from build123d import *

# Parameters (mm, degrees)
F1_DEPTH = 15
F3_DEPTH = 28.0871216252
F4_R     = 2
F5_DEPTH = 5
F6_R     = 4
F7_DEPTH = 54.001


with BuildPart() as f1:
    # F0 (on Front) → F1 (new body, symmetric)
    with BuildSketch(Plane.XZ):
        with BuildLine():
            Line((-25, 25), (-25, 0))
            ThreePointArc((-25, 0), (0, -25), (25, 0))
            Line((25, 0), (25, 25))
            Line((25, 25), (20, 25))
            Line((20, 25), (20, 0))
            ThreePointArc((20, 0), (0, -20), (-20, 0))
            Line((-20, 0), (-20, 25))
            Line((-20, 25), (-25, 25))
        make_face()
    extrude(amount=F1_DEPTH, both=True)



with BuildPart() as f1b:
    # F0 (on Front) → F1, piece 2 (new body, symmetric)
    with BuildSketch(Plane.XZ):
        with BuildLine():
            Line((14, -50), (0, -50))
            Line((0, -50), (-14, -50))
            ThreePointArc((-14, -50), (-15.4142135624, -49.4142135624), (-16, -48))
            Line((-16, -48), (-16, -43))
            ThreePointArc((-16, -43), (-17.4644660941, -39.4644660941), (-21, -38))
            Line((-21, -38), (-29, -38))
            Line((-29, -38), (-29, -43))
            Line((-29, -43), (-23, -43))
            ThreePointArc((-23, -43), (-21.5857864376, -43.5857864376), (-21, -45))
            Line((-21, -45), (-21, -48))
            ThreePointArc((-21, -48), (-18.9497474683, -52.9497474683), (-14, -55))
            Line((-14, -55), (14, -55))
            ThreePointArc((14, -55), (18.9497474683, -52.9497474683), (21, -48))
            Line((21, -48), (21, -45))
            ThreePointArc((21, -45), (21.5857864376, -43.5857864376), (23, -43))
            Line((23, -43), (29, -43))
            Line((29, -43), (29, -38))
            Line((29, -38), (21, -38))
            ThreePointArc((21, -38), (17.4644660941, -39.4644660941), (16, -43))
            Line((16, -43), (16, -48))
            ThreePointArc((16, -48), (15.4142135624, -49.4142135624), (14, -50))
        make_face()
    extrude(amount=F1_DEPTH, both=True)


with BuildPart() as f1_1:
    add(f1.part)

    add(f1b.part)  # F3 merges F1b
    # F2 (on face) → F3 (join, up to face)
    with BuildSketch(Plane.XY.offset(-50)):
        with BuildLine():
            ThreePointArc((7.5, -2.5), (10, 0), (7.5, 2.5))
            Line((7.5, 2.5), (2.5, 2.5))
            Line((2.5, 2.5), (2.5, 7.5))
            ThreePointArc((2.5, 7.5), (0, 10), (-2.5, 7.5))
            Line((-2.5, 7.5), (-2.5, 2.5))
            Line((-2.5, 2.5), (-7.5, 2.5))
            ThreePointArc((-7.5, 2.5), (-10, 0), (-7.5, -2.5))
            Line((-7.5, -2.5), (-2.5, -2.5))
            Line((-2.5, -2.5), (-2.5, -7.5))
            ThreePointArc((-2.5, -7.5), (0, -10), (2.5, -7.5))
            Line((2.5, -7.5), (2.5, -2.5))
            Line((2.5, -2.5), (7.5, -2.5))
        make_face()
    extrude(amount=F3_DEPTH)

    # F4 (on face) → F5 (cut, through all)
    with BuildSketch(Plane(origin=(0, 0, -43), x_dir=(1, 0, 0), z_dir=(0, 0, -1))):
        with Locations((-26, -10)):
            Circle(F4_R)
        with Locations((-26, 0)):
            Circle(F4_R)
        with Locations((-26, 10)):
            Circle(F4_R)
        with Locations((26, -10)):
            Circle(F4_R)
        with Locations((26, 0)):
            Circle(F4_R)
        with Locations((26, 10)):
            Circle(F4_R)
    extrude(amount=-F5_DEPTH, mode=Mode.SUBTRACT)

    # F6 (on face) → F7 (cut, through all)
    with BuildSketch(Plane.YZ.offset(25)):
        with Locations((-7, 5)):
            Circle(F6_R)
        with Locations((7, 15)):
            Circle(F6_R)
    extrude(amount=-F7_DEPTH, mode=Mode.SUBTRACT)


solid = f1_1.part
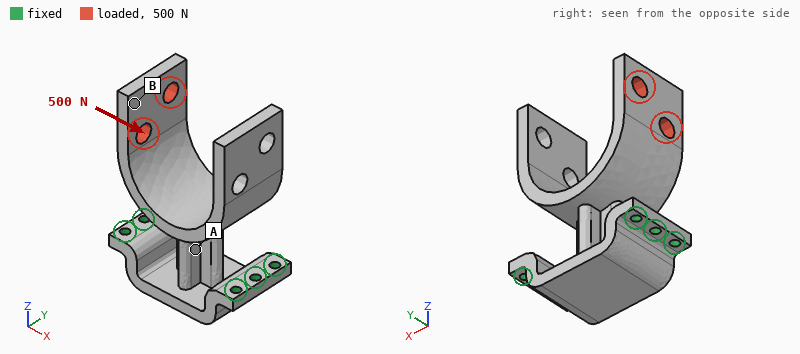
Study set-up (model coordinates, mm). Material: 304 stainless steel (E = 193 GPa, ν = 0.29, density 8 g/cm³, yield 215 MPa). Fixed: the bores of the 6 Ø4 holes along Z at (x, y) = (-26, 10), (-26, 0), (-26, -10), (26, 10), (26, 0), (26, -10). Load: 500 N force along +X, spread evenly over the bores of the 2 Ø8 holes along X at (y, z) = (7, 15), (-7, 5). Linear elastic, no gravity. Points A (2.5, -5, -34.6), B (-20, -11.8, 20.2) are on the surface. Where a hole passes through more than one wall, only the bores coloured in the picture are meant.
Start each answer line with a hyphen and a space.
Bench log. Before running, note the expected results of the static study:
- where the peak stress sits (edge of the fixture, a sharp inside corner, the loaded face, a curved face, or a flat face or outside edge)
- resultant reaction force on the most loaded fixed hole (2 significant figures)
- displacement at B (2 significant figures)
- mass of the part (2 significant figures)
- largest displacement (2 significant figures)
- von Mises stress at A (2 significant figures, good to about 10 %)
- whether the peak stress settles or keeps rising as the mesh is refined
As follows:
- a sharp inside corner
- 330 N
- 0.36 mm
- 260 g
- 0.42 mm
- 24 MPa
- keeps rising
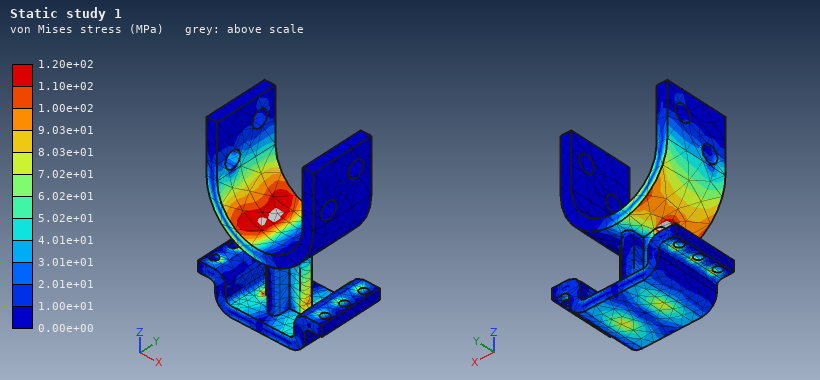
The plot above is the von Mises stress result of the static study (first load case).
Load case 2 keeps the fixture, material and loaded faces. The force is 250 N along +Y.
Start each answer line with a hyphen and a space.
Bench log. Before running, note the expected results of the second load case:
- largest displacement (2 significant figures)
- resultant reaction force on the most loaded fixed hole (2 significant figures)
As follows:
- 0.16 mm
- 400 N
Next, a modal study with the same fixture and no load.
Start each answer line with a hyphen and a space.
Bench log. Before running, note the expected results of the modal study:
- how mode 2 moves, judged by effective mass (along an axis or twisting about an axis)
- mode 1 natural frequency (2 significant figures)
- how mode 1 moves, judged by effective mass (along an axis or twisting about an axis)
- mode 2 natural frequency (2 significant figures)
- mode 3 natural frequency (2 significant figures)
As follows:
- along Y
- 850 Hz
- along X
- 910 Hz
- 1400 Hz
